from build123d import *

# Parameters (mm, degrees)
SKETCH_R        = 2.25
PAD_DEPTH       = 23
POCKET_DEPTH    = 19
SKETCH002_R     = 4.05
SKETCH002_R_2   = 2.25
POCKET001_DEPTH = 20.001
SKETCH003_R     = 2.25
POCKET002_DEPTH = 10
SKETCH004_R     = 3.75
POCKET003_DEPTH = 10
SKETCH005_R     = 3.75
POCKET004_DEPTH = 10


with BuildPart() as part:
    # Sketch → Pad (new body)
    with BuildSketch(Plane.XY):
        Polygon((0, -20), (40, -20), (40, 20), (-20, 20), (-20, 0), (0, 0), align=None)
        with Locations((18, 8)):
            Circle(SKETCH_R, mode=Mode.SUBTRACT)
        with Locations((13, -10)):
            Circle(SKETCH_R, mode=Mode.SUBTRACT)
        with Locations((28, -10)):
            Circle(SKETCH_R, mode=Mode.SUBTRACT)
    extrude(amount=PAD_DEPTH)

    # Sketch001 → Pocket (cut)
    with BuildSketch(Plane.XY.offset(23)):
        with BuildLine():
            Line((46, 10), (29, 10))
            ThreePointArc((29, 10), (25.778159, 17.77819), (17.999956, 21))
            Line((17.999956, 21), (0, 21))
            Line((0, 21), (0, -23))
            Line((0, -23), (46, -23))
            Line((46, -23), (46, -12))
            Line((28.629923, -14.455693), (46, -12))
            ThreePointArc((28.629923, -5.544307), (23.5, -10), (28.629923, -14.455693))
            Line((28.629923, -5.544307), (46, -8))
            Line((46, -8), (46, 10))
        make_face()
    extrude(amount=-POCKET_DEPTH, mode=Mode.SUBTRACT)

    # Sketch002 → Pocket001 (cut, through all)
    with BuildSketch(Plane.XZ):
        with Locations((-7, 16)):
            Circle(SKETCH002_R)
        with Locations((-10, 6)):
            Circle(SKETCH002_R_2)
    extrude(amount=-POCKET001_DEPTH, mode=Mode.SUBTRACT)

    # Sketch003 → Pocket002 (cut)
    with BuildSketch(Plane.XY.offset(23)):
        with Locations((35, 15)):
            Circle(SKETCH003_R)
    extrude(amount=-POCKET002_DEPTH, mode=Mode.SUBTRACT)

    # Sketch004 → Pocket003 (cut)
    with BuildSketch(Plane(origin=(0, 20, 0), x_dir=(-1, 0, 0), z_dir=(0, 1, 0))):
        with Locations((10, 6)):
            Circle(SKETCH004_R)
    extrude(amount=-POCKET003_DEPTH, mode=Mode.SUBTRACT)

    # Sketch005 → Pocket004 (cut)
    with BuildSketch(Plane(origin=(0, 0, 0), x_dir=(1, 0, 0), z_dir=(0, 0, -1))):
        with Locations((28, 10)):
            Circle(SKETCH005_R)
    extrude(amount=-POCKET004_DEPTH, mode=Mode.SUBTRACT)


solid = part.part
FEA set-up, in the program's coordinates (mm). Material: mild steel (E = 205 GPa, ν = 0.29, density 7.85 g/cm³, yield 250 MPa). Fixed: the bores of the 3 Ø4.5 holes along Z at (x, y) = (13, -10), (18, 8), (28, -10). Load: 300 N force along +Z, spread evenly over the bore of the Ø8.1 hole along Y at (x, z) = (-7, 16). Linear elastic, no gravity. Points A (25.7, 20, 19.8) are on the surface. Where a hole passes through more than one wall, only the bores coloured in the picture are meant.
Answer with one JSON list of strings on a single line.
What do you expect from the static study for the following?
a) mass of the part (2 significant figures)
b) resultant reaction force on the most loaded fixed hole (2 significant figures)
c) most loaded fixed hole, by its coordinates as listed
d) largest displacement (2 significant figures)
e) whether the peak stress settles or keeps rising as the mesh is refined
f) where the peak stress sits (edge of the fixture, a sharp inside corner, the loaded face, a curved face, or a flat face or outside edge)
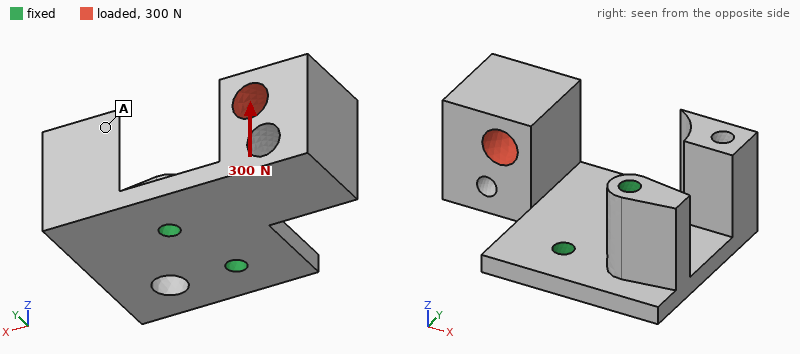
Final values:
["140 g", "230 N", "(18, 8)", "0.10 mm", "keeps rising", "edge of the fixture"]
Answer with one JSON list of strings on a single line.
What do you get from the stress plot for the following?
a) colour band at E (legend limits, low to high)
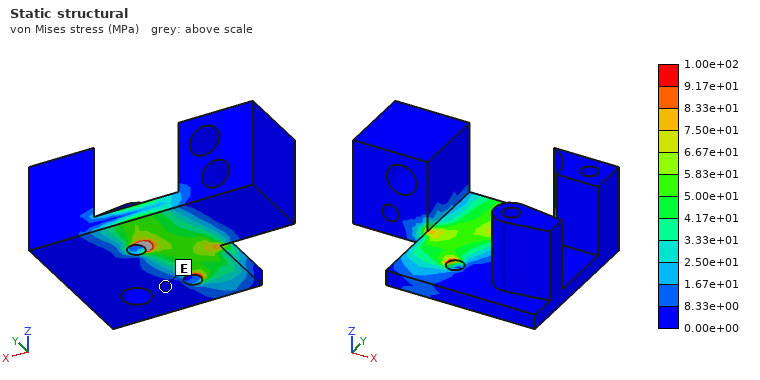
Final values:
["0.00e+00 to 8.33e+00 MPa"]
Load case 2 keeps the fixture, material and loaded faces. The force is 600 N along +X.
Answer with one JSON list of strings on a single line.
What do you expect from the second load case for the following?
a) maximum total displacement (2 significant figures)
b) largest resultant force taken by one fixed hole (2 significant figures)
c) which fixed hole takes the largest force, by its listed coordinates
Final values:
["0.19 mm", "620 N", "(18, 8)"]
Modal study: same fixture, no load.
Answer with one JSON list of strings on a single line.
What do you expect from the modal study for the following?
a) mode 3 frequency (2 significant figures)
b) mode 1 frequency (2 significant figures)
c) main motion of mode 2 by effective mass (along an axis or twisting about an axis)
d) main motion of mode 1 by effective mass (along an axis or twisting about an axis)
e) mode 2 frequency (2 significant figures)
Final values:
["3400 Hz", "1200 Hz", "along Y", "along Z", "3000 Hz"]
